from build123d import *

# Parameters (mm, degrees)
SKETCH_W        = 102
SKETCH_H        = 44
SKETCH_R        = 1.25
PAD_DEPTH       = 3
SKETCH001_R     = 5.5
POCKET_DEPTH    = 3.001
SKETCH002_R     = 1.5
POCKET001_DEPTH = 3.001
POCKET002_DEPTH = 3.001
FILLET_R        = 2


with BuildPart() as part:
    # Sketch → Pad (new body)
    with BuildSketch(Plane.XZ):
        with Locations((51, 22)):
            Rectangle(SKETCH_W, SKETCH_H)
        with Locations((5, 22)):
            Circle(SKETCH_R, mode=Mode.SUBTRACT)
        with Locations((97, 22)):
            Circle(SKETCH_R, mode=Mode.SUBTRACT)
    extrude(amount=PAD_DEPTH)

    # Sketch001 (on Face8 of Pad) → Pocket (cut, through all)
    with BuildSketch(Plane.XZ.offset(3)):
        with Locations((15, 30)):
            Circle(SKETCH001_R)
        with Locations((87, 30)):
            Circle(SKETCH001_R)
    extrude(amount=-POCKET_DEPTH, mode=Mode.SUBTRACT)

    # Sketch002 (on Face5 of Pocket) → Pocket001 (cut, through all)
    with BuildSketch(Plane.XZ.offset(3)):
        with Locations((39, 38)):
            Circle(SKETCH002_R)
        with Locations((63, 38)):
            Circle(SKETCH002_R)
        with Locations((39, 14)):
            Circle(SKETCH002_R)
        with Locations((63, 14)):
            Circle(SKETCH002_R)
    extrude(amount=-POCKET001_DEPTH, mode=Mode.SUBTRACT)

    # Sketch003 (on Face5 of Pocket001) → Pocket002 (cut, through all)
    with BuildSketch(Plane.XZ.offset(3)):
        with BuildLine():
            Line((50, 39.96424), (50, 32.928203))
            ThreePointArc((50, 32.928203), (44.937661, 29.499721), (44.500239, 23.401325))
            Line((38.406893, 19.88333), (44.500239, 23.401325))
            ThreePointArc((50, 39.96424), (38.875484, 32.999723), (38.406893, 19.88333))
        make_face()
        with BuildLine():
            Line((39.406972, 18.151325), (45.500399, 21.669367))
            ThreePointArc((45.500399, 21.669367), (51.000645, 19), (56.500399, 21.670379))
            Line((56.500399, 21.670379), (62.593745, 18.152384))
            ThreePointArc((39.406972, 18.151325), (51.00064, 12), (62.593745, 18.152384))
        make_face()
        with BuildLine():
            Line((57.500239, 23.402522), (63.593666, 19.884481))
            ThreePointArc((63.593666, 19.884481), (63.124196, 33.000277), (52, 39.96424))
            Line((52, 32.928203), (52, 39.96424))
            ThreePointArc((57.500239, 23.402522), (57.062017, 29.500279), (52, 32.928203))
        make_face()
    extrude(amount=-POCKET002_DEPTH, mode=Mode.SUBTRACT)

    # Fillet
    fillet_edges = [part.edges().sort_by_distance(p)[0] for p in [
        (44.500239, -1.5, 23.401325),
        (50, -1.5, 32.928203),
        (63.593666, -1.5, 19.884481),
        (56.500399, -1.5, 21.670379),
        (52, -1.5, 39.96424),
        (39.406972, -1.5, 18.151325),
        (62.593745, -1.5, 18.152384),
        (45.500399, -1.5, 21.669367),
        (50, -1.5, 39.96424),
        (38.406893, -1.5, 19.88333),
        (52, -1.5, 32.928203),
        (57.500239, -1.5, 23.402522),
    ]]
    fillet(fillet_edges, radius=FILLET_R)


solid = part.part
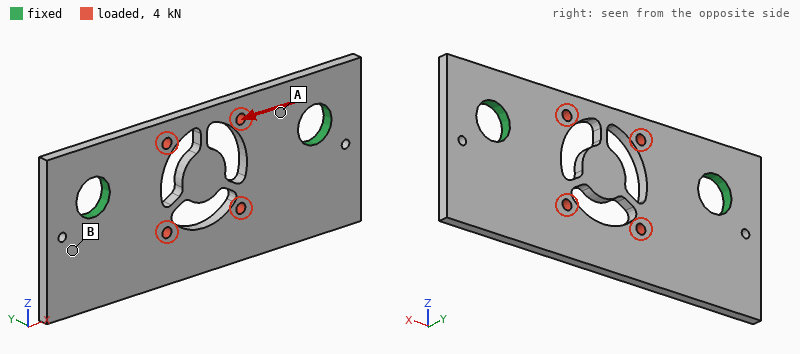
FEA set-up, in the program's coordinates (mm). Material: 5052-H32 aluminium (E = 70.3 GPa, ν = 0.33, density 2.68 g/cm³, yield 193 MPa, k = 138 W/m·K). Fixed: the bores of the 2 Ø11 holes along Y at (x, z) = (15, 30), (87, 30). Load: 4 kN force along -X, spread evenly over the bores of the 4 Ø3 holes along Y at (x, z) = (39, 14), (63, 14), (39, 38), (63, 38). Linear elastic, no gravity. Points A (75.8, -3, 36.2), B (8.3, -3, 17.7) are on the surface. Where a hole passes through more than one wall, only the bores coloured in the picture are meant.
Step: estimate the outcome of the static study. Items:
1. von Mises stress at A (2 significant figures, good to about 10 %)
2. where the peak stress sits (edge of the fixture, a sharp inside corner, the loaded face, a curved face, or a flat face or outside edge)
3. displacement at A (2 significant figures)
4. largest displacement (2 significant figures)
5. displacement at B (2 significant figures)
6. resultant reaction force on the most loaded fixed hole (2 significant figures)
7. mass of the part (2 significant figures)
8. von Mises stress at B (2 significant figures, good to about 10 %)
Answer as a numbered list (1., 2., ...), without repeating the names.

1. 27 MPa
2. the loaded face
3. 3.0 µm
4. 16 µm
5. 4.7 µm
6. 2.0 kN
7. 31 g
8. 8.3 MPa
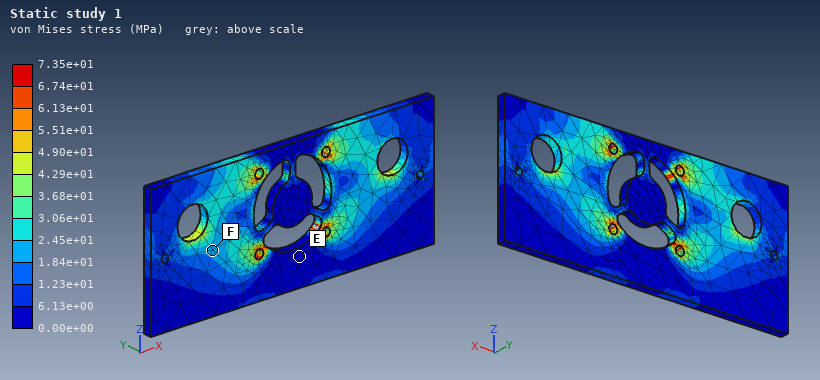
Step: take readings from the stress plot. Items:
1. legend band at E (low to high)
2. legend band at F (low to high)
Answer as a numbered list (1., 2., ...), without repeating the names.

1. 0.00e+00 to 6.13e+00 MPa
2. 1.84e+01 to 2.45e+01 MPa
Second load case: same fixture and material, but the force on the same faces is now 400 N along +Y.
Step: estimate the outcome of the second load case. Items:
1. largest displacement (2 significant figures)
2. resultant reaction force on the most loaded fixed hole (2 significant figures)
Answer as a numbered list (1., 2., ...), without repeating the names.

1. 0.11 mm
2. 200 N
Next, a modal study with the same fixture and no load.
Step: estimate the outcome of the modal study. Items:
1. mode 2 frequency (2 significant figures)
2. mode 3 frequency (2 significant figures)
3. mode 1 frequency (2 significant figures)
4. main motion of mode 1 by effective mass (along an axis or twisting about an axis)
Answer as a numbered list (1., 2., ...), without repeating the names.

1. 3900 Hz
2. 4000 Hz
3. 2500 Hz
4. along Y
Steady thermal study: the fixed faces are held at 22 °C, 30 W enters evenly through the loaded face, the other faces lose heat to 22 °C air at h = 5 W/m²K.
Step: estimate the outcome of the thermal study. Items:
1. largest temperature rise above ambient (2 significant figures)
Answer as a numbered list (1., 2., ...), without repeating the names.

1. 29 K
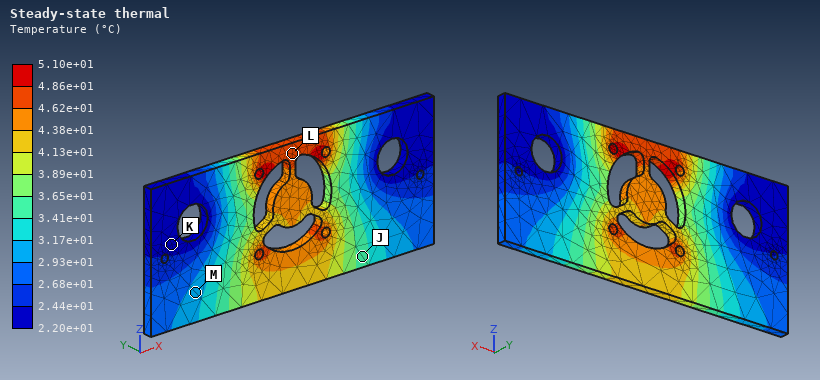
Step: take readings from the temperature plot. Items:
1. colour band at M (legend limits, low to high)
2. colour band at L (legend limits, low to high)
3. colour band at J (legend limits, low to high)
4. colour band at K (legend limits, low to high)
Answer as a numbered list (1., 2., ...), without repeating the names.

1. 2.93e+01 to 3.17e+01 °C
2. 4.62e+01 to 4.86e+01 °C
3. 3.41e+01 to 3.65e+01 °C
4. 2.20e+01 to 2.44e+01 °C
